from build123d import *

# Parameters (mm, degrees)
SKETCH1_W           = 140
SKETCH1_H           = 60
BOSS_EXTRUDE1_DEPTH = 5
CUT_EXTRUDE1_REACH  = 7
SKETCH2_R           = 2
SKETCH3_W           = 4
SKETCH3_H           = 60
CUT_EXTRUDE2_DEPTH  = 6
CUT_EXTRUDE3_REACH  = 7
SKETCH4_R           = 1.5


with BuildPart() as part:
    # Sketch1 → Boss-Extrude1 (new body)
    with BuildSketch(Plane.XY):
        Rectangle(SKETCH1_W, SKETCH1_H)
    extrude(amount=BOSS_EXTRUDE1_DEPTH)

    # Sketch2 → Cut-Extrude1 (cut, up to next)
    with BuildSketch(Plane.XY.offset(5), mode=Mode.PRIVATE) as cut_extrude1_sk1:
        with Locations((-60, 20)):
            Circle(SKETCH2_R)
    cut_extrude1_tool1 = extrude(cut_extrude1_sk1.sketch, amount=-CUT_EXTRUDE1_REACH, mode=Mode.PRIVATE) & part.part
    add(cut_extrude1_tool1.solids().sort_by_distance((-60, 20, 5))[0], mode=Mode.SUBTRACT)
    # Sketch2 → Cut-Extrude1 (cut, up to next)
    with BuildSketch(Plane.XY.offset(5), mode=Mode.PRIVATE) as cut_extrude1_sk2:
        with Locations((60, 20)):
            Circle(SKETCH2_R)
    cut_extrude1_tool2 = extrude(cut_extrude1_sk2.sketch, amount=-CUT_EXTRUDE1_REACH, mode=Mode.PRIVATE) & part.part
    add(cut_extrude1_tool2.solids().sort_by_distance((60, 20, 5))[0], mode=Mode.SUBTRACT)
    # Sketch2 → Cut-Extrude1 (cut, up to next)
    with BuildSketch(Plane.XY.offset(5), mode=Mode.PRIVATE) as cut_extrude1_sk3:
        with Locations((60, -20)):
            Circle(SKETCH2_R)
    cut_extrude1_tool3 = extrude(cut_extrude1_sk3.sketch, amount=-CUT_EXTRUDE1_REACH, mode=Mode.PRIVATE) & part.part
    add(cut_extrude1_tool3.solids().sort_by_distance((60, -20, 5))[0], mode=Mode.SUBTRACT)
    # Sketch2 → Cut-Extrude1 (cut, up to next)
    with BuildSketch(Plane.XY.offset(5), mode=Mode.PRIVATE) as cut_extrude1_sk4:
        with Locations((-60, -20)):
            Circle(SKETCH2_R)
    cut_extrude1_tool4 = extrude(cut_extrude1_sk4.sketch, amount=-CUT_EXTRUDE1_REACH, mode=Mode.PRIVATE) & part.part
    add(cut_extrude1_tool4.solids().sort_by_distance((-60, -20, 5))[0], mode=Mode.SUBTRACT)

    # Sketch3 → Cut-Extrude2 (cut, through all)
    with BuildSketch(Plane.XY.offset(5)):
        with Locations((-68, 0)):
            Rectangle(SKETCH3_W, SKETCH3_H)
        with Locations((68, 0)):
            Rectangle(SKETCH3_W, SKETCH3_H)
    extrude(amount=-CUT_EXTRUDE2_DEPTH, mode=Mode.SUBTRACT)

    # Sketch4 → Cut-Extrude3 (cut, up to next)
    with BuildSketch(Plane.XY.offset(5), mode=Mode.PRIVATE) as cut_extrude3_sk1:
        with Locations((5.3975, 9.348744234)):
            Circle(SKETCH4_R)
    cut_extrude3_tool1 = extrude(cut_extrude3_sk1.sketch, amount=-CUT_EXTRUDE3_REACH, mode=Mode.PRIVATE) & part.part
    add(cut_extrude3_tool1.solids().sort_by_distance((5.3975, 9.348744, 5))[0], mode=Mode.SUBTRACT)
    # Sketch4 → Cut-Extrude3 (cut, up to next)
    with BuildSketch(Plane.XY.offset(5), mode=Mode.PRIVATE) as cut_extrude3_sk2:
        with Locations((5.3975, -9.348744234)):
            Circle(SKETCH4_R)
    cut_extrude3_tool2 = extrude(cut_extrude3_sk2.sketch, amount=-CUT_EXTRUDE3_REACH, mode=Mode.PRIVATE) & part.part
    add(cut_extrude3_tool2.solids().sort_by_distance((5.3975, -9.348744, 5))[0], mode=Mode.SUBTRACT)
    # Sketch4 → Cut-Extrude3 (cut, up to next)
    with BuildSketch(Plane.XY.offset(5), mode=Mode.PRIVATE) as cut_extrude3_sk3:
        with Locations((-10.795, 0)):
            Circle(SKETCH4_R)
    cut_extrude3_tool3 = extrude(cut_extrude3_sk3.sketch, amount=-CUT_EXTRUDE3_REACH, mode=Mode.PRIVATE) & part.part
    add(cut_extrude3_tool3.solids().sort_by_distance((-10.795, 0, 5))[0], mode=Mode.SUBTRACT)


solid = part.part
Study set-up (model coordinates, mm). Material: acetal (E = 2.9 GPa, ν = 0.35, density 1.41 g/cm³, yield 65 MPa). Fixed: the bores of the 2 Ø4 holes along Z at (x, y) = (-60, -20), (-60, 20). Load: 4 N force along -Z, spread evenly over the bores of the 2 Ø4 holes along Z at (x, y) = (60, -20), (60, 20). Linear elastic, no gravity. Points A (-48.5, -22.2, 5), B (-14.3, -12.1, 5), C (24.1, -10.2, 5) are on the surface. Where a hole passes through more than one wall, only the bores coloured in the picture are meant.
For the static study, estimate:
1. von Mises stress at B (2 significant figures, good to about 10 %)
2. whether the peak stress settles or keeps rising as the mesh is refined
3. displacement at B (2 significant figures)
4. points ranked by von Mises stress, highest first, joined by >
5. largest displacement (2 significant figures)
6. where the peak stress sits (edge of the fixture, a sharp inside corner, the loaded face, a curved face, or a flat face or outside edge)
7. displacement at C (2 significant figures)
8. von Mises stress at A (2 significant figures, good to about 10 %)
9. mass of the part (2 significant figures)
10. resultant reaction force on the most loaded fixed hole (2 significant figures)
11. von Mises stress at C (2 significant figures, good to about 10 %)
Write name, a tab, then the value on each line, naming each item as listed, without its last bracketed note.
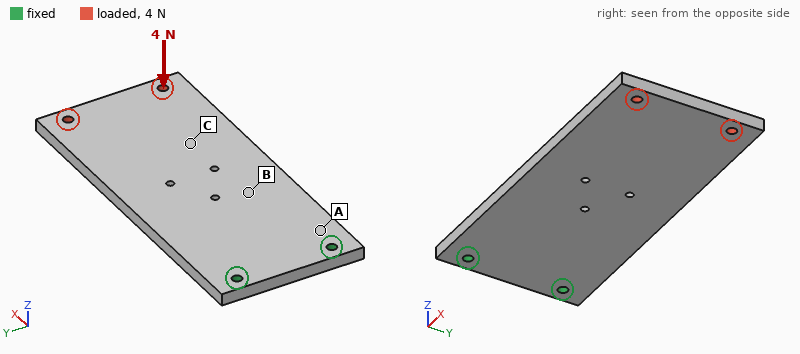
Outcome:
von Mises stress at B	1.2 MPa
whether the peak stress settles or keeps rising as the mesh is refined	keeps rising
displacement at B	0.28 mm
points ranked by von Mises stress, highest first, joined by >	A > B > C
largest displacement	1.5 mm
where the peak stress sits	edge of the fixture
displacement at C	0.78 mm
von Mises stress at A	1.8 MPa
mass of the part	55 g
resultant reaction force on the most loaded fixed hole	2.0 N
von Mises stress at C	0.58 MPa
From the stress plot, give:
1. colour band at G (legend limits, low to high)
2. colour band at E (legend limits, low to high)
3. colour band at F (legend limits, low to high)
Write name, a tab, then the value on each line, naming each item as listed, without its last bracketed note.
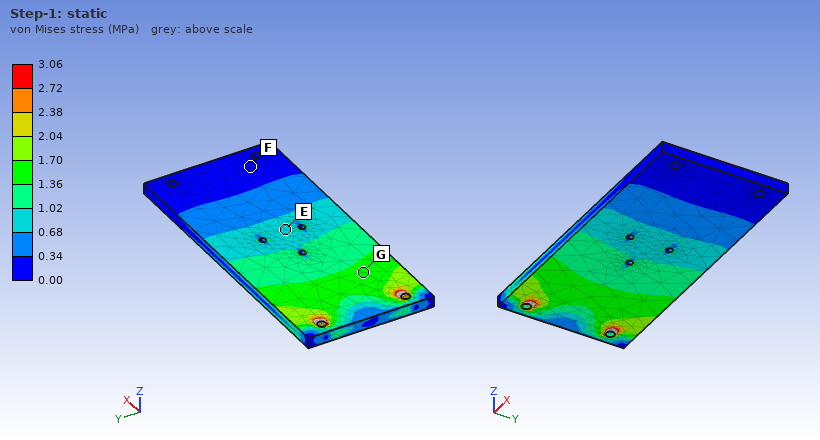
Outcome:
colour band at G	1.36 to 1.70 MPa
colour band at E	0.68 to 1.02 MPa
colour band at F	0.00 to 0.34 MPa
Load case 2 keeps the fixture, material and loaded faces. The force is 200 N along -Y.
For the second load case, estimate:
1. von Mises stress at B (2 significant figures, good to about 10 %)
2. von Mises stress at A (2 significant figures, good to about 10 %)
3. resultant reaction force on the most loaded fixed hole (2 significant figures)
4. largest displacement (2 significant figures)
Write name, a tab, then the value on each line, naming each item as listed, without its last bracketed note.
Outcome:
von Mises stress at B	2.5 MPa
von Mises stress at A	6.4 MPa
resultant reaction force on the most loaded fixed hole	580 N
largest displacement	0.68 mm
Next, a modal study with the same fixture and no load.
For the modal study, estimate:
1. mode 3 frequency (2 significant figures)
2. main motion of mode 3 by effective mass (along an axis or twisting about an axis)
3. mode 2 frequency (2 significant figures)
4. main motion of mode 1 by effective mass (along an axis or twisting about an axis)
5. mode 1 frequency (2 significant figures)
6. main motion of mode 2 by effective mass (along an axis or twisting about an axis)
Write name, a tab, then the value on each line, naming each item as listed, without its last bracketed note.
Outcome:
mode 3 frequency	440 Hz
main motion of mode 3 by effective mass	along Z
mode 2 frequency	320 Hz
main motion of mode 1 by effective mass	along Z
mode 1 frequency	71 Hz
main motion of mode 2 by effective mass	twisting about X
